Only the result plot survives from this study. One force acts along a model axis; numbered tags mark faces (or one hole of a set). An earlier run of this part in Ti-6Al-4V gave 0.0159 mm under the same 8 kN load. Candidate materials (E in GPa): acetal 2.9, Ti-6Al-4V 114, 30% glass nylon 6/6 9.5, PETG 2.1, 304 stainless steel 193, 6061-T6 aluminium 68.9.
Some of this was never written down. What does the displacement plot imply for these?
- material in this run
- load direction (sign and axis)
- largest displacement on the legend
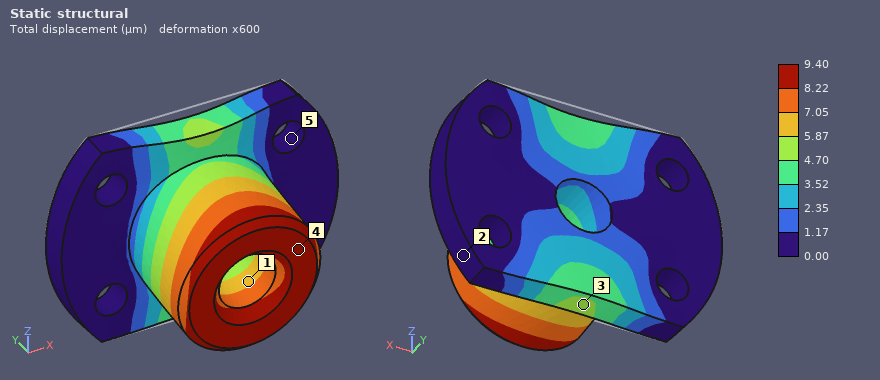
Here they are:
304 stainless steel
-Z
9.40 µm
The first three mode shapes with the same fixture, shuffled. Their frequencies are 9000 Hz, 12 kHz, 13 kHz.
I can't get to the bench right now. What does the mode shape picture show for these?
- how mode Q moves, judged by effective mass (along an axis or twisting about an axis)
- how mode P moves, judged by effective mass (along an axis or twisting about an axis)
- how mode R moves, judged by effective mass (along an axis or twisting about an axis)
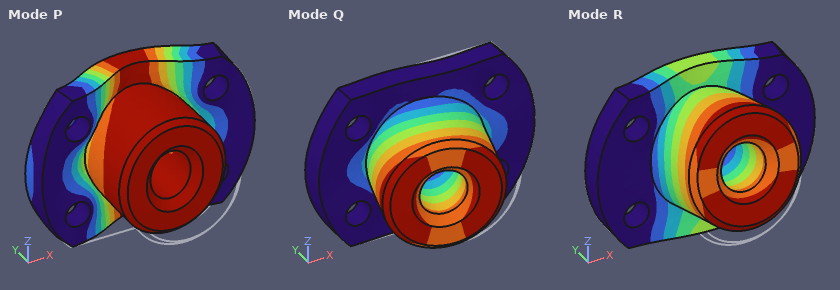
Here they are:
along X
along Y
along Z
